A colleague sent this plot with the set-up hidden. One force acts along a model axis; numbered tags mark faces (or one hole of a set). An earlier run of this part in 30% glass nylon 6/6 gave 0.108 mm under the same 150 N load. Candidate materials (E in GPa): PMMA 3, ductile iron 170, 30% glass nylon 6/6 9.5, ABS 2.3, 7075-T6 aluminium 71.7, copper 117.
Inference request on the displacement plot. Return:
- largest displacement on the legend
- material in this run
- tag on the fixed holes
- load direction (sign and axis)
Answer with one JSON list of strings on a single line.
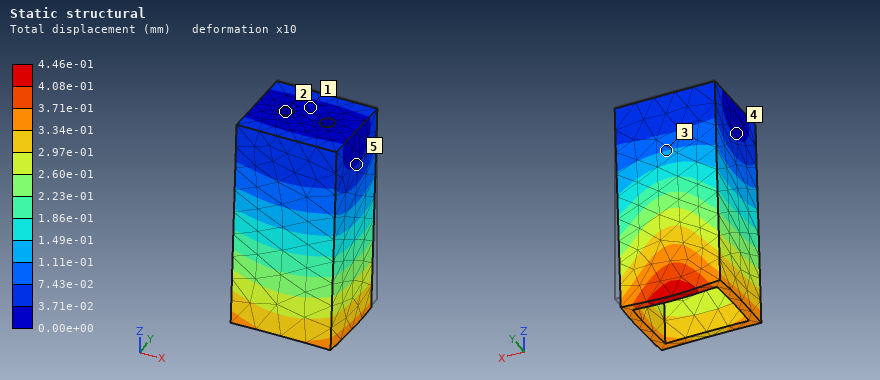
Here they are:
["4.46e-01 mm", "ABS", "2", "-Y"]
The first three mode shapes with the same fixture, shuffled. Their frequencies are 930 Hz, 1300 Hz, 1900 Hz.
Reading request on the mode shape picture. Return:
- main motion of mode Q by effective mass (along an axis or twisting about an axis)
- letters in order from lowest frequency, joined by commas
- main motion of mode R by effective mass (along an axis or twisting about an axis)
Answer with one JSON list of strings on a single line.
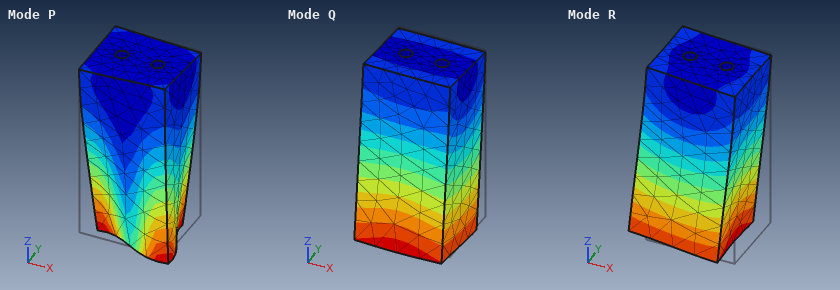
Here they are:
["along Y", "Q, R, P", "along X"]
